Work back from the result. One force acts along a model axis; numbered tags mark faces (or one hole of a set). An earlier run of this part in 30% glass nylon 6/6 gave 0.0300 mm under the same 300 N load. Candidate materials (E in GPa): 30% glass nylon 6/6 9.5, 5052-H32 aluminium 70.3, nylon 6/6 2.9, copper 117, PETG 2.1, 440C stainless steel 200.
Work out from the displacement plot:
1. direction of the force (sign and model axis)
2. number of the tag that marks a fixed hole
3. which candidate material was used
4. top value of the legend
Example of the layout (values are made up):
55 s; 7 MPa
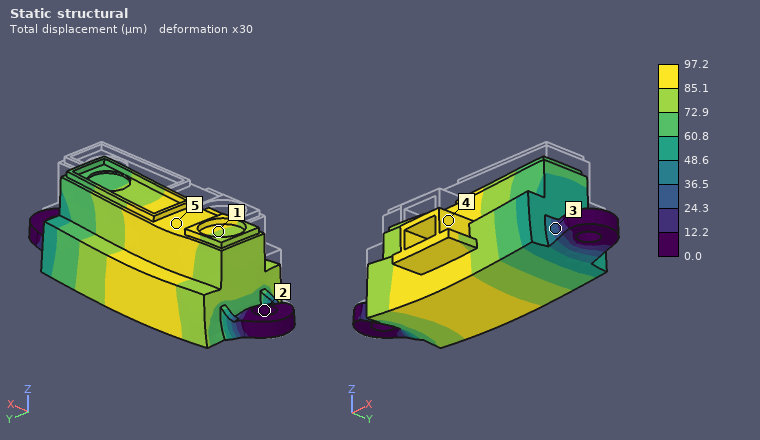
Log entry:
-Z; 2; nylon 6/6; 97.2 µm
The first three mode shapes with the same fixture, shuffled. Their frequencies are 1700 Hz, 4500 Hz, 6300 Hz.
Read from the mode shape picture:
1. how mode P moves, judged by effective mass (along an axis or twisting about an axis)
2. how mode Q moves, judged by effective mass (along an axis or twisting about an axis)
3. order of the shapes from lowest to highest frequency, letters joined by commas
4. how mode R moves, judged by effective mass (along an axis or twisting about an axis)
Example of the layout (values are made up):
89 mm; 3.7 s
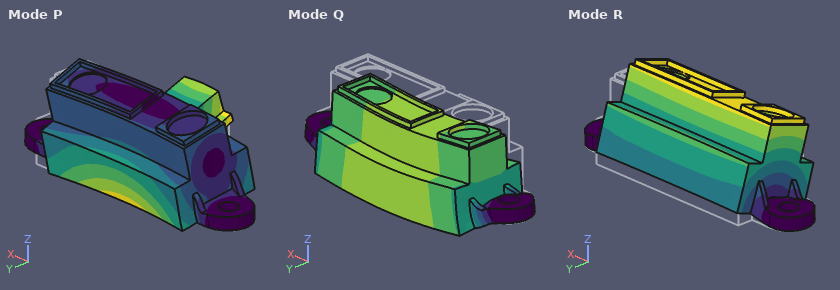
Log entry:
along Y; along Z; R, Q, P; along Y
